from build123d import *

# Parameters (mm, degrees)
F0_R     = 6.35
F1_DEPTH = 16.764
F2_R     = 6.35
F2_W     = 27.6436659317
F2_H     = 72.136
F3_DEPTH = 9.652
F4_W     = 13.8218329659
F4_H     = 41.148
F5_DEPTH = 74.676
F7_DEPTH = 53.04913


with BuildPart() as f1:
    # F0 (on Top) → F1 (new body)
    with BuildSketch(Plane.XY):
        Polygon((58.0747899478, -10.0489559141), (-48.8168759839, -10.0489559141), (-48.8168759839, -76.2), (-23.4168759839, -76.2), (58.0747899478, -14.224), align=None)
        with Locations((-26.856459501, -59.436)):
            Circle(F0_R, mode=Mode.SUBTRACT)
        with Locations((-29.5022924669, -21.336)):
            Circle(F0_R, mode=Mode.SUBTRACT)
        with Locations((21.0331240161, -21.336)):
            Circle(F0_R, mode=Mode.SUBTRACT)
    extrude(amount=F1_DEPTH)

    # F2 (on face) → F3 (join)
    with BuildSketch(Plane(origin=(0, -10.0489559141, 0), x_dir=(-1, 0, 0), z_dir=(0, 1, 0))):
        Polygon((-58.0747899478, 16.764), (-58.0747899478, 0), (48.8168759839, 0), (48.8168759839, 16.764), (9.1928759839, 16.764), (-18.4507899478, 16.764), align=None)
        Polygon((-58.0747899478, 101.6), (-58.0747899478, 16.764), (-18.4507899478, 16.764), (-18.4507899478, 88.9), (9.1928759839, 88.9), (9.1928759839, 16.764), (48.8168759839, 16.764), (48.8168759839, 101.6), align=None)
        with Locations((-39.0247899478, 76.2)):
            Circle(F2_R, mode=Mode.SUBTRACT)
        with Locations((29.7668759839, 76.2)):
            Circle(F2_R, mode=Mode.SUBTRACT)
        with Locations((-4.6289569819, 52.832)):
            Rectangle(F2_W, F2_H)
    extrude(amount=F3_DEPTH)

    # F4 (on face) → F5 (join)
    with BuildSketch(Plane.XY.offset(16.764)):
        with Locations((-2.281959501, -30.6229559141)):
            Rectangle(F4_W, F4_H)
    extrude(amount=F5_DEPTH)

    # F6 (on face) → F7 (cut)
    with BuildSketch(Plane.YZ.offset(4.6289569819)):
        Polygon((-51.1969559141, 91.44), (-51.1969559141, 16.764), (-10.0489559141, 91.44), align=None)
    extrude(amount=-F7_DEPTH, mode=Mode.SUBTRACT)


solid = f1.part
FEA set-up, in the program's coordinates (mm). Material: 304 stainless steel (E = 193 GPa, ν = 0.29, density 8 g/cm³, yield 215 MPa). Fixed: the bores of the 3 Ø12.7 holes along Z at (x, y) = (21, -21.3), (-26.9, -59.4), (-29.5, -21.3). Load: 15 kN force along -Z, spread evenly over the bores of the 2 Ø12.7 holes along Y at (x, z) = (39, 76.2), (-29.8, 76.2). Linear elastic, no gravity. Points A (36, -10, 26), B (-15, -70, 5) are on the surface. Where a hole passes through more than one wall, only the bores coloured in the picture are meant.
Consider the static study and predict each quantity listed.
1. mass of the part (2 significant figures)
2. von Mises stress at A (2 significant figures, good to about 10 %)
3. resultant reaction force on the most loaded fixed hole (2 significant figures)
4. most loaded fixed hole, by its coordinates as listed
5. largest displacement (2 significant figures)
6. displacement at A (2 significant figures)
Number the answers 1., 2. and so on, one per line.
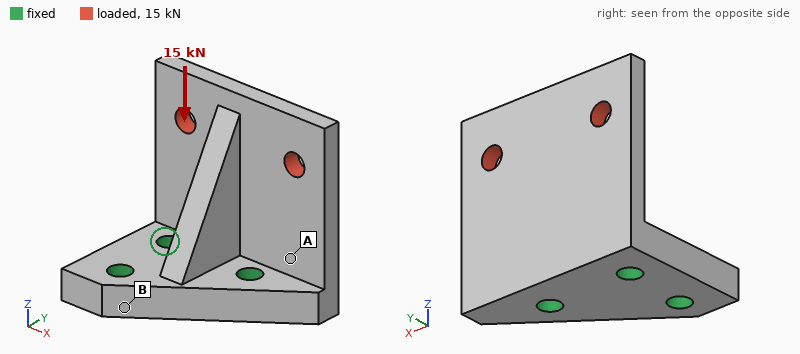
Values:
1. 1.5 kg
2. 21 MPa
3. 9.9 kN
4. (21, -21.3)
5. 28 µm
6. 8.4 µm
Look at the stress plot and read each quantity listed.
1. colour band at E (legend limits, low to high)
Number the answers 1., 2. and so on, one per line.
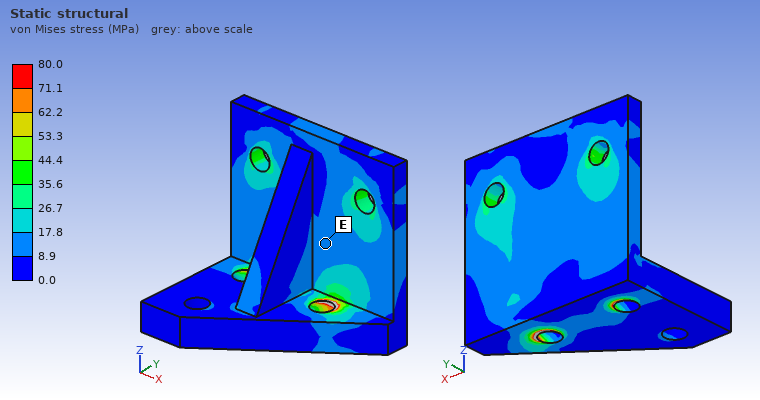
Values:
1. 8.9 to 17.8 MPa
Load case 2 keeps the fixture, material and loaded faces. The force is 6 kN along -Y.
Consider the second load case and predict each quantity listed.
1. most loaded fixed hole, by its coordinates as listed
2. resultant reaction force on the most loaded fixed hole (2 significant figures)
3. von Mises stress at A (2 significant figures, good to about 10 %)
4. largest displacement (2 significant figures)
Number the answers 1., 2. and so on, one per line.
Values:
1. (-26.9, -59.4)
2. 5.2 kN
3. 33 MPa
4. 0.16 mm
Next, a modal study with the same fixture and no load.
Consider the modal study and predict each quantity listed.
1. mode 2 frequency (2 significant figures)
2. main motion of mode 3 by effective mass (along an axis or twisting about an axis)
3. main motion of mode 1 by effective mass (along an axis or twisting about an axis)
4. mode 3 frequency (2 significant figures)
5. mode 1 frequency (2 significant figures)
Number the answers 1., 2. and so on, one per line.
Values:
1. 2600 Hz
2. along X
3. along Y
4. 3800 Hz
5. 2100 Hz
